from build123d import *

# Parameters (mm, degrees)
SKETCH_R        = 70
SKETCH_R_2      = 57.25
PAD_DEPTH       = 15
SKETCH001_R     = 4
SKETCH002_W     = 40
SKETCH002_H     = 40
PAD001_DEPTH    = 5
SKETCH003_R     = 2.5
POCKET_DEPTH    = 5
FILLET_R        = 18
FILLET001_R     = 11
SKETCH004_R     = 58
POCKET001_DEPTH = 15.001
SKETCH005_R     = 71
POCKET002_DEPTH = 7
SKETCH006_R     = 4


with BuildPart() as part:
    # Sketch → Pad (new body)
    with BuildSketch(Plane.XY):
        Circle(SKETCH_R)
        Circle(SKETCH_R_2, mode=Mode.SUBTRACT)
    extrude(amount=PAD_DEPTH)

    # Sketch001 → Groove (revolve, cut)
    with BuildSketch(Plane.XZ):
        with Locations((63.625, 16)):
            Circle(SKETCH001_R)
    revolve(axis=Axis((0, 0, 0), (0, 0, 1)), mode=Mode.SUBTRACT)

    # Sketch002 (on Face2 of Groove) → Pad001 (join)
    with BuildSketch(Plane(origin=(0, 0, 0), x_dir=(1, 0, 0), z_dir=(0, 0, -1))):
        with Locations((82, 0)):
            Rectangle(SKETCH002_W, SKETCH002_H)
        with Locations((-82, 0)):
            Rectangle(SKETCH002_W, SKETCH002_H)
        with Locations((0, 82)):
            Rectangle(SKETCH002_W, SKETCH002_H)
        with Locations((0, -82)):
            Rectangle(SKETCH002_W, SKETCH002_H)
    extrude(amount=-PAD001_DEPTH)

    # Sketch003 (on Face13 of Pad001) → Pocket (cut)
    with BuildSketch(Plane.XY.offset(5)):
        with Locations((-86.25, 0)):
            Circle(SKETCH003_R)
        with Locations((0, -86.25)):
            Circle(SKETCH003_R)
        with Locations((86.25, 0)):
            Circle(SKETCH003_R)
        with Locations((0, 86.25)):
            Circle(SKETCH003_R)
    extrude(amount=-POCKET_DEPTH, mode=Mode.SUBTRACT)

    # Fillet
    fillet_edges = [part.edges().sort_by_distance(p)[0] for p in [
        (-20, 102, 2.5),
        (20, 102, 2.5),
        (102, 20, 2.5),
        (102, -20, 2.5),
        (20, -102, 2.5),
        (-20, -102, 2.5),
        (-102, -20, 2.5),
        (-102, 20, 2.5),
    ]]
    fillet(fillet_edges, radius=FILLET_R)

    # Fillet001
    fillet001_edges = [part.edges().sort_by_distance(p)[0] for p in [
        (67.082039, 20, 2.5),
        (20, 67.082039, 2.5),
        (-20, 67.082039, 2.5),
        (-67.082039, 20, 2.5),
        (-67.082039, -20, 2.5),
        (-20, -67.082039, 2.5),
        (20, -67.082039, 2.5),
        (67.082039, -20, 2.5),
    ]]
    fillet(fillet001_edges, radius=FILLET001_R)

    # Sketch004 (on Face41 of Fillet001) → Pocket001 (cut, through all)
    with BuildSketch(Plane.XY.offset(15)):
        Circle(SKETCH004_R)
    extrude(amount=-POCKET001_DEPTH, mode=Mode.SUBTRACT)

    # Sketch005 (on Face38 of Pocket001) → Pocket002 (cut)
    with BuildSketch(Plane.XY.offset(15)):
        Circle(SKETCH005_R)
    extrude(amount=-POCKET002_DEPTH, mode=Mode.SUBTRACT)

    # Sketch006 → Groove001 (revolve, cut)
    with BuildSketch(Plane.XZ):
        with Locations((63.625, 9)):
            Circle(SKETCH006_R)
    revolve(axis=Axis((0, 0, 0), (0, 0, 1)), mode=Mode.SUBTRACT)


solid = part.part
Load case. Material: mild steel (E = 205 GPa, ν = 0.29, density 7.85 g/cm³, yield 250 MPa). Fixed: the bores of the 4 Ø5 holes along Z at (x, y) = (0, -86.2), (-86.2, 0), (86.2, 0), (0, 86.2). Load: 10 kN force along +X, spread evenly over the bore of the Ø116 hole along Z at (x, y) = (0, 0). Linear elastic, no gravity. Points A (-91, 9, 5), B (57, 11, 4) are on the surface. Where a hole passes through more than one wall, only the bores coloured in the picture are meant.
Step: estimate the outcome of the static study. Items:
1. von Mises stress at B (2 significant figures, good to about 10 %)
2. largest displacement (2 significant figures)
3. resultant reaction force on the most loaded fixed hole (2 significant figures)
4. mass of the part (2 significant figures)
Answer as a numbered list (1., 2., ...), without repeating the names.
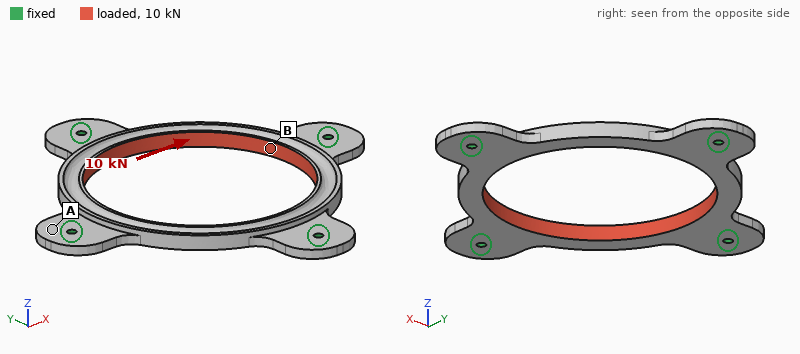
1. 52 MPa
2. 35 µm
3. 2.6 kN
4. 430 g
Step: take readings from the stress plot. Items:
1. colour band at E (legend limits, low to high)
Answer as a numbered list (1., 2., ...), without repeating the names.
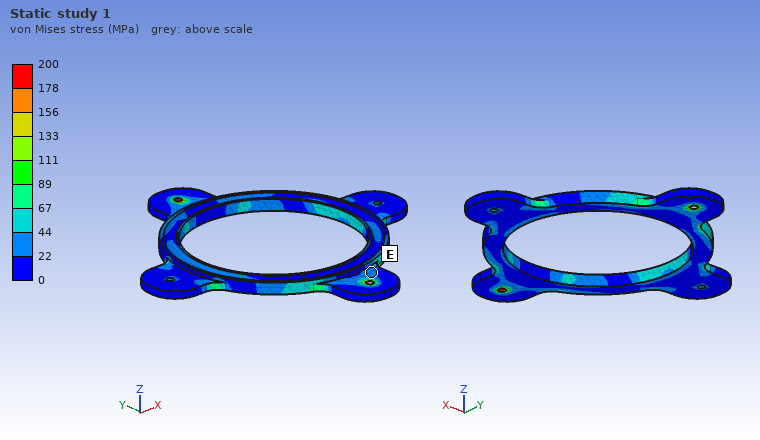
1. 22 to 44 MPa
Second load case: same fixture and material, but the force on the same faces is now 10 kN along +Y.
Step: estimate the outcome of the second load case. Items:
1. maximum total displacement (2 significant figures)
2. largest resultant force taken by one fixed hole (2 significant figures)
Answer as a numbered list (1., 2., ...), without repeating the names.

1. 35 µm
2. 2.6 kN
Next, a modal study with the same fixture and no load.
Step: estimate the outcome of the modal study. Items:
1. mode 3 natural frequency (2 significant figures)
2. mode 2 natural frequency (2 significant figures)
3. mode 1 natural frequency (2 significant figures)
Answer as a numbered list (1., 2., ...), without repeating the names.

1. 2400 Hz
2. 2300 Hz
3. 2300 Hz
